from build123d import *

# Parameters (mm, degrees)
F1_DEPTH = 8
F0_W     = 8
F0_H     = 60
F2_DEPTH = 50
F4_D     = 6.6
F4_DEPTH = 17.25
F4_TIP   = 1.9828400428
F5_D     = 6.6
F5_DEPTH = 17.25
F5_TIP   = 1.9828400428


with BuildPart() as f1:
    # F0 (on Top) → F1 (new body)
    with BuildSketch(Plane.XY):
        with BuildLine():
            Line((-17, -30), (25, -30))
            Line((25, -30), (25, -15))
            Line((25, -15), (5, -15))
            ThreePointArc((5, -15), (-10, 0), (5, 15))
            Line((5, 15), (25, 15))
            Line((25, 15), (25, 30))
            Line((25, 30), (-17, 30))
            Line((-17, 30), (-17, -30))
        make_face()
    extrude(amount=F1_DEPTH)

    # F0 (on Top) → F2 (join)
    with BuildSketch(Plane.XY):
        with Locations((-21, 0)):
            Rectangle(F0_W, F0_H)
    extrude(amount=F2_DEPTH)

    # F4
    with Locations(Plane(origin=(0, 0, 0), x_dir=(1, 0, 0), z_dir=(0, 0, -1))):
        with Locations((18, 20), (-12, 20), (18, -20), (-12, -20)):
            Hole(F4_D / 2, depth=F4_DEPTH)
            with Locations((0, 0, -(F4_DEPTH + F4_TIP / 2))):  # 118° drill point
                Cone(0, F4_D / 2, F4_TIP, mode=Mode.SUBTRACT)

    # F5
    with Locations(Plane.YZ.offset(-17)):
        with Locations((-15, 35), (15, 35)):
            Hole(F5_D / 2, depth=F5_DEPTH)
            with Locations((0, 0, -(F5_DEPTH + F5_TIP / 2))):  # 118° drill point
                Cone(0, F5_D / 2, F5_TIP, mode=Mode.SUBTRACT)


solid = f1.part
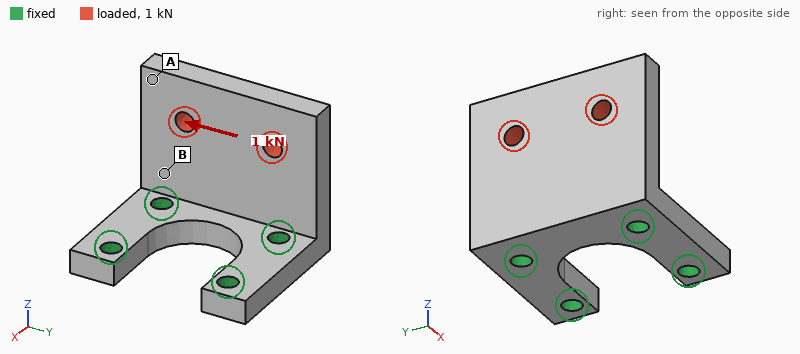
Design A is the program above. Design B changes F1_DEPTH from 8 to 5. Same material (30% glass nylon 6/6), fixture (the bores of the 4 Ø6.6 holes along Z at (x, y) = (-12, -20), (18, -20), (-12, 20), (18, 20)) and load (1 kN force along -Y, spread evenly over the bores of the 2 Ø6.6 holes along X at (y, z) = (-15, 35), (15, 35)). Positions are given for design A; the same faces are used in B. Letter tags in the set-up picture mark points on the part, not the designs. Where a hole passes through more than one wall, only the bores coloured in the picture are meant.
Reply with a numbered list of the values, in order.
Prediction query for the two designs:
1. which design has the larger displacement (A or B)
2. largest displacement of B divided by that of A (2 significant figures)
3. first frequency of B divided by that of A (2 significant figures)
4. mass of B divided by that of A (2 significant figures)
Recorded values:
1. B
2. 1.8
3. 0.64
4. 0.88
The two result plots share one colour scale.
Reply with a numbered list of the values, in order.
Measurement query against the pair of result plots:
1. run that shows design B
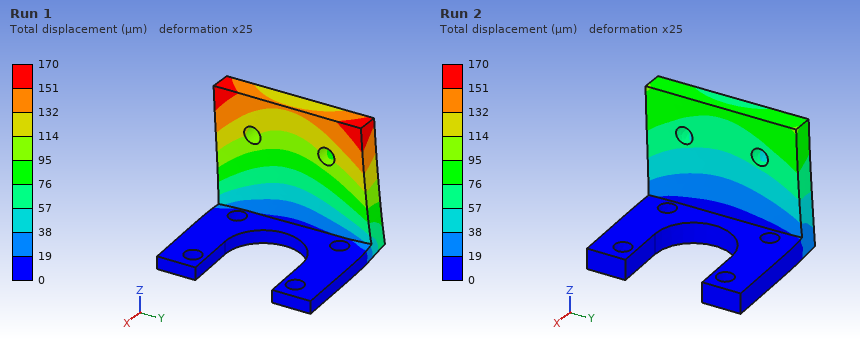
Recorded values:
1. Run 1
